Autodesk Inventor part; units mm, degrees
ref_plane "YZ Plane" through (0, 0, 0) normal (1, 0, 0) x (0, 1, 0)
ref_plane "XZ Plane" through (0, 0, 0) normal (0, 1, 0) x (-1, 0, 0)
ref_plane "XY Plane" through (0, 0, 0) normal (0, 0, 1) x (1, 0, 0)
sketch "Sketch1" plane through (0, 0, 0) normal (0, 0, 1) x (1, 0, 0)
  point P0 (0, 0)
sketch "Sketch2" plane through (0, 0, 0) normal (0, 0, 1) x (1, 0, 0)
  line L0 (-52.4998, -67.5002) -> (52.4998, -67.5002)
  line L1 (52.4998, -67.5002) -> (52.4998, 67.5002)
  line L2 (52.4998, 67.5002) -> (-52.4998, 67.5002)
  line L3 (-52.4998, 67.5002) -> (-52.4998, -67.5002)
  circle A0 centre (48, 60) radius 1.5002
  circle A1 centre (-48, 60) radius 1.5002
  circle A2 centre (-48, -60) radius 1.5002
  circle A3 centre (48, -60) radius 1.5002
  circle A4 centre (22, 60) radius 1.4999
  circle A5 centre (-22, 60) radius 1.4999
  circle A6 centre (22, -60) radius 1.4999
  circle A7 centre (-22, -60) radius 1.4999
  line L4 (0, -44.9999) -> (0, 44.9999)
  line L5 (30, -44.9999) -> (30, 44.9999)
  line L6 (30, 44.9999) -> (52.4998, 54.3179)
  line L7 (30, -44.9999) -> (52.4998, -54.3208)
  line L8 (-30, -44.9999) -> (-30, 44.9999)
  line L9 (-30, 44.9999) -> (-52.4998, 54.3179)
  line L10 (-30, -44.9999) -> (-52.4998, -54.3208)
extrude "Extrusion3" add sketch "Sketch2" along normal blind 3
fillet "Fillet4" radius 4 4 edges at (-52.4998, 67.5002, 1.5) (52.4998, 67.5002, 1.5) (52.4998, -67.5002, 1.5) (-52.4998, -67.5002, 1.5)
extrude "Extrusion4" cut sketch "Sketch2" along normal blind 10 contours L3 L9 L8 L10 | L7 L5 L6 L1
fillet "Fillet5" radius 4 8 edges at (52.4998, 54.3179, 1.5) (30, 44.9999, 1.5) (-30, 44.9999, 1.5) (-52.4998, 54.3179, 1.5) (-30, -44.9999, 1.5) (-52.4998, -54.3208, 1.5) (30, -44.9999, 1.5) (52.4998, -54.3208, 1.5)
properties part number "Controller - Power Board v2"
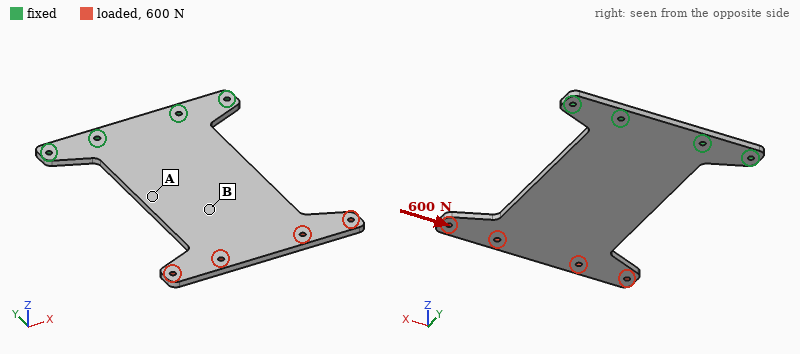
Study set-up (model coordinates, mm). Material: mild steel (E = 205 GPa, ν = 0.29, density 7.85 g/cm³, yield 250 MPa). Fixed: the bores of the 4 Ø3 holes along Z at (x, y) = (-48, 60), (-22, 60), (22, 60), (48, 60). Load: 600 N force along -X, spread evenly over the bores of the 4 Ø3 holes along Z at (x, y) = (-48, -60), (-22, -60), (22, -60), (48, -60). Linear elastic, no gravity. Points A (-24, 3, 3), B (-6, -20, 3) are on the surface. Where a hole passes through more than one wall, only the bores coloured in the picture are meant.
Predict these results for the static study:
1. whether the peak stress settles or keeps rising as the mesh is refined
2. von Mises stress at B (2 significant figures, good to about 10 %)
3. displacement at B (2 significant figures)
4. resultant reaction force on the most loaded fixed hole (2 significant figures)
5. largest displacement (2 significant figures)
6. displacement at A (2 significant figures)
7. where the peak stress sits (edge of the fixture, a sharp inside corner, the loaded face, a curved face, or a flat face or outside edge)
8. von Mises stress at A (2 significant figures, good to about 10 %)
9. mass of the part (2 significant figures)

keeps rising
8.8 MPa
19 µm
1.1 kN
44 µm
12 µm
edge of the fixture
17 MPa
230 g
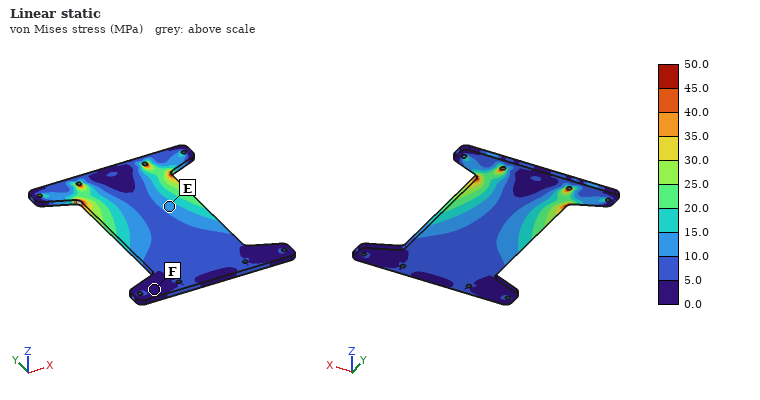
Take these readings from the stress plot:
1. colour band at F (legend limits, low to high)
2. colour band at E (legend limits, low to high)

0.0 to 5.0 MPa
10.0 to 15.0 MPa
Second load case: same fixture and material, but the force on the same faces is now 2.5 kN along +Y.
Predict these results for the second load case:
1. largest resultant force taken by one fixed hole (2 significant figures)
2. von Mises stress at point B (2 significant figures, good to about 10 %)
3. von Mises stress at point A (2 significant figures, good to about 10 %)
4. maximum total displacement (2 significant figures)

1.2 kN
11 MPa
14 MPa
26 µm
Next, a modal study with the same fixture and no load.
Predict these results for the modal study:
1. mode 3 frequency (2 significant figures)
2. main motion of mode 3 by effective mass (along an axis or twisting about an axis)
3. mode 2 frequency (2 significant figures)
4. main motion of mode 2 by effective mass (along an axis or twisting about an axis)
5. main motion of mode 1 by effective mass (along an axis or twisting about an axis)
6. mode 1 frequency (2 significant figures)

880 Hz
along Z
470 Hz
twisting about Y
along Z
130 Hz
